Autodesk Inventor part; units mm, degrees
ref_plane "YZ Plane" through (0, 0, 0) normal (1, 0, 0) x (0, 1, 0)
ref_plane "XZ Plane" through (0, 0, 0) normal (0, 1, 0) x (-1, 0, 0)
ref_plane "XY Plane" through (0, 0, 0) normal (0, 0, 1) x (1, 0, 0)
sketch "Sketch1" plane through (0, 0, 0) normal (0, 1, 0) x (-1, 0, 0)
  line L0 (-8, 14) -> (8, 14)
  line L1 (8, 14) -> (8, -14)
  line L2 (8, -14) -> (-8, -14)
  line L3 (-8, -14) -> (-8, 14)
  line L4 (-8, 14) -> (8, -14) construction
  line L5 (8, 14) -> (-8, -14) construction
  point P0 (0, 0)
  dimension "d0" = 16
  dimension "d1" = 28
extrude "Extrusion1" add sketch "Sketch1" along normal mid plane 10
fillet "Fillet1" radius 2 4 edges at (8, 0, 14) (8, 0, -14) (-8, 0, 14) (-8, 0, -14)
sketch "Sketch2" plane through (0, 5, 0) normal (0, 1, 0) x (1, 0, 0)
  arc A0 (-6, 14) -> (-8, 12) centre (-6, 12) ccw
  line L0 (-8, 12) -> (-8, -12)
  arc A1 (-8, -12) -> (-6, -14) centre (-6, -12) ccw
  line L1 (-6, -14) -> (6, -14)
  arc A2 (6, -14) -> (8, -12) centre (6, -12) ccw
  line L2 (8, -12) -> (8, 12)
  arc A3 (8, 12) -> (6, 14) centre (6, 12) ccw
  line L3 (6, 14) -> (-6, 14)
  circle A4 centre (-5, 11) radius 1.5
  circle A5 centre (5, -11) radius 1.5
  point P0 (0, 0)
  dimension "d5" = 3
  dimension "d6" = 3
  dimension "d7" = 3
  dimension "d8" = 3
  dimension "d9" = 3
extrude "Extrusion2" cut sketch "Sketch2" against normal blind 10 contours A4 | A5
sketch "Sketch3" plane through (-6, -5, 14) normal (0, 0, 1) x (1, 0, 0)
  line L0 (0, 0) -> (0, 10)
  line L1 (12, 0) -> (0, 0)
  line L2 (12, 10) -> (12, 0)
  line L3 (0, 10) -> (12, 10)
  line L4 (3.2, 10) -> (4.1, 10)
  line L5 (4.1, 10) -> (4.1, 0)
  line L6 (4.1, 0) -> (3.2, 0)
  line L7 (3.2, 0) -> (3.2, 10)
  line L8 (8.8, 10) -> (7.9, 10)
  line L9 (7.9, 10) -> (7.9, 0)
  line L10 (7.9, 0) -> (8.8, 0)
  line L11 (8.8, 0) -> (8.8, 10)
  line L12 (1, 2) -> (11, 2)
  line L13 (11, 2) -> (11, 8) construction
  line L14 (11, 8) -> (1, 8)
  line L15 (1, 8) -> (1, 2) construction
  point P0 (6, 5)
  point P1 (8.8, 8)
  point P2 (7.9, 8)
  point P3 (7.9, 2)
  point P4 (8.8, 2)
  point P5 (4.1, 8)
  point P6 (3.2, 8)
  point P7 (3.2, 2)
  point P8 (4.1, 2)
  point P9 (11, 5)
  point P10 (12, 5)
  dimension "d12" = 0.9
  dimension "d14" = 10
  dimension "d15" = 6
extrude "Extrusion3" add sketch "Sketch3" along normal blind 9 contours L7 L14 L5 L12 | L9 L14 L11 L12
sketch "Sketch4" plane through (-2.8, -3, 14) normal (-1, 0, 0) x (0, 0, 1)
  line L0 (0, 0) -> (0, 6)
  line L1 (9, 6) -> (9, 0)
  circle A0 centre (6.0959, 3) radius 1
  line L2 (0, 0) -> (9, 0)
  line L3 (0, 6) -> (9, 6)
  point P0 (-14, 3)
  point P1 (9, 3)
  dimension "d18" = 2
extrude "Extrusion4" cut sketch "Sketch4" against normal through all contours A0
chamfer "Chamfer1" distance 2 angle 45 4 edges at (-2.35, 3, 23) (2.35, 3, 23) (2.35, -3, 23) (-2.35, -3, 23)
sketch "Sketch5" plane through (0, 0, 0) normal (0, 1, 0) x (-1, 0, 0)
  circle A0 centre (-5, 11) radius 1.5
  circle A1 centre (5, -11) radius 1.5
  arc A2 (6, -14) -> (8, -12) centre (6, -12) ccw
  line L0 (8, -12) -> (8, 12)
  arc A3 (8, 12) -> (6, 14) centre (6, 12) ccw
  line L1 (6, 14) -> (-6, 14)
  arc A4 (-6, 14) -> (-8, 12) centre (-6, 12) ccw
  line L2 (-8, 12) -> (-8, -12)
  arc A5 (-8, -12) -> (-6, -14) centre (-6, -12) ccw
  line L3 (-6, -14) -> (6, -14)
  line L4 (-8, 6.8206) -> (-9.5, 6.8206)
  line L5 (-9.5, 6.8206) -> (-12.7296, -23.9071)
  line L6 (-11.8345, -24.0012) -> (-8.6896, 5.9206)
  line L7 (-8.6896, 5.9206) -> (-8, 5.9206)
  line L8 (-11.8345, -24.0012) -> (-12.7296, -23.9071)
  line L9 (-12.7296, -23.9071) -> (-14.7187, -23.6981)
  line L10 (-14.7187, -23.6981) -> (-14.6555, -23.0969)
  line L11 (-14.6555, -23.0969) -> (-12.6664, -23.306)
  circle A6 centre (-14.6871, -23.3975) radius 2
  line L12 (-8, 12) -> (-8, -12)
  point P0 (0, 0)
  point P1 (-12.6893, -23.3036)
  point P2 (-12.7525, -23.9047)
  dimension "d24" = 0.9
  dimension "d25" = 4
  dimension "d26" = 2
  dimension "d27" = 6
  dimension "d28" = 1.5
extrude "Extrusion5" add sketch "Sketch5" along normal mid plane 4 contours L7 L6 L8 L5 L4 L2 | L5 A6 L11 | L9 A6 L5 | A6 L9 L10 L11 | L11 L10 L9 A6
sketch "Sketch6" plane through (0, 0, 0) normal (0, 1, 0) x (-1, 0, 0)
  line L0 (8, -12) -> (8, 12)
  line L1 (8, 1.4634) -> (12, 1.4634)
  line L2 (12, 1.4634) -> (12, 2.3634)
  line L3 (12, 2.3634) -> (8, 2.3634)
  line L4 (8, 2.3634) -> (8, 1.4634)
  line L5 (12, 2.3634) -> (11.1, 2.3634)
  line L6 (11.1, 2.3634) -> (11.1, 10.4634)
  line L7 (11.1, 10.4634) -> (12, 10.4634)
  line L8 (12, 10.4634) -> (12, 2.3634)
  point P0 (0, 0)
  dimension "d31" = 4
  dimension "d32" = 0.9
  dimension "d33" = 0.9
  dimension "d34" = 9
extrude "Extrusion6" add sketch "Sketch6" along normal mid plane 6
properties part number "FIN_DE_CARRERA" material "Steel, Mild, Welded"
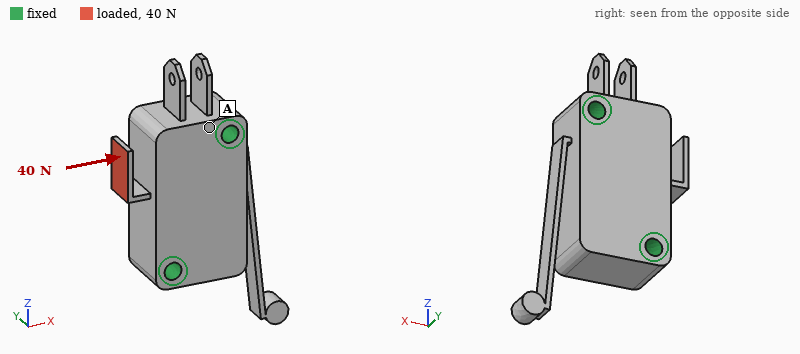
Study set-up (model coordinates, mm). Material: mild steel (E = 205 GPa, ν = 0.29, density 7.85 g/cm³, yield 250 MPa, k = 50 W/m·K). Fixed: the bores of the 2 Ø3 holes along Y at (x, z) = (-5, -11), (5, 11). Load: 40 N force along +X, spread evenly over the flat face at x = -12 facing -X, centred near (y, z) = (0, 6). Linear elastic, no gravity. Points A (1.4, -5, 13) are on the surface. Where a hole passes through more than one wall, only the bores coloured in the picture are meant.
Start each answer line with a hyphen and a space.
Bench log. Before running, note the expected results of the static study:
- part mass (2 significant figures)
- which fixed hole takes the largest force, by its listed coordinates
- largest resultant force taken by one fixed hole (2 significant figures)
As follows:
- 36 g
- (5, 11)
- 32 N
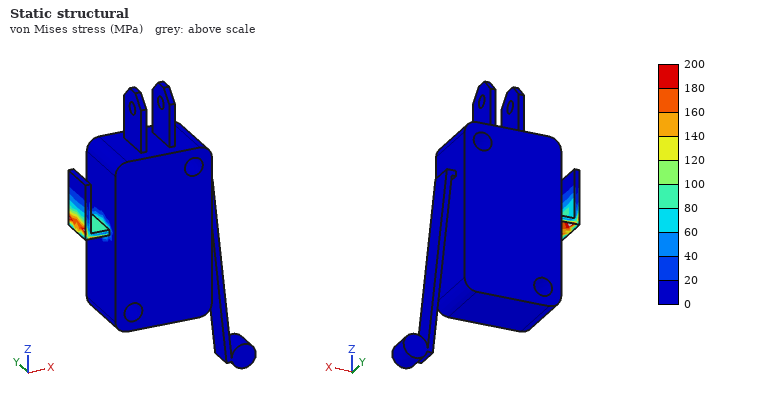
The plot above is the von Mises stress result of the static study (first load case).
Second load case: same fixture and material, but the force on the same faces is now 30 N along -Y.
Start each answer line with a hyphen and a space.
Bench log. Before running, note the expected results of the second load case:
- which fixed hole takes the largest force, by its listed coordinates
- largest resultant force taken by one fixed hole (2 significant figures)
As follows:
- (5, 11)
- 16 N
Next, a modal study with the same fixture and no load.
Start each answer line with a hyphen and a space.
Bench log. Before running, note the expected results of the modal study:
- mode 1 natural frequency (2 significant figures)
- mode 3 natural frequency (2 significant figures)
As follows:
- 450 Hz
- 3400 Hz
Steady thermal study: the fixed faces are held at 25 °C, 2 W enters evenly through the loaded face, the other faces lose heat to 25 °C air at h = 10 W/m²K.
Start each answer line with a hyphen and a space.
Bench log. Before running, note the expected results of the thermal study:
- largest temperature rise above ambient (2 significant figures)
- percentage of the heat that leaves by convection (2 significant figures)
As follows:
- 59 K
- 3.2 %
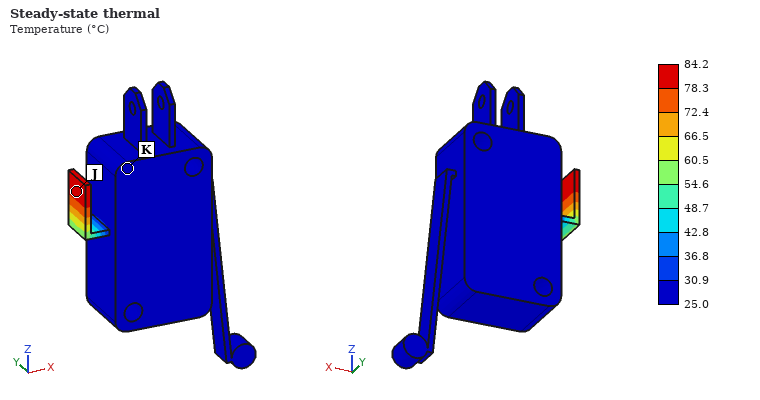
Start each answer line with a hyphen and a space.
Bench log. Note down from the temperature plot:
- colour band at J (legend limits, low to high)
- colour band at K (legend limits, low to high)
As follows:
- 78.3 to 84.2 °C
- 25.0 to 30.9 °C
